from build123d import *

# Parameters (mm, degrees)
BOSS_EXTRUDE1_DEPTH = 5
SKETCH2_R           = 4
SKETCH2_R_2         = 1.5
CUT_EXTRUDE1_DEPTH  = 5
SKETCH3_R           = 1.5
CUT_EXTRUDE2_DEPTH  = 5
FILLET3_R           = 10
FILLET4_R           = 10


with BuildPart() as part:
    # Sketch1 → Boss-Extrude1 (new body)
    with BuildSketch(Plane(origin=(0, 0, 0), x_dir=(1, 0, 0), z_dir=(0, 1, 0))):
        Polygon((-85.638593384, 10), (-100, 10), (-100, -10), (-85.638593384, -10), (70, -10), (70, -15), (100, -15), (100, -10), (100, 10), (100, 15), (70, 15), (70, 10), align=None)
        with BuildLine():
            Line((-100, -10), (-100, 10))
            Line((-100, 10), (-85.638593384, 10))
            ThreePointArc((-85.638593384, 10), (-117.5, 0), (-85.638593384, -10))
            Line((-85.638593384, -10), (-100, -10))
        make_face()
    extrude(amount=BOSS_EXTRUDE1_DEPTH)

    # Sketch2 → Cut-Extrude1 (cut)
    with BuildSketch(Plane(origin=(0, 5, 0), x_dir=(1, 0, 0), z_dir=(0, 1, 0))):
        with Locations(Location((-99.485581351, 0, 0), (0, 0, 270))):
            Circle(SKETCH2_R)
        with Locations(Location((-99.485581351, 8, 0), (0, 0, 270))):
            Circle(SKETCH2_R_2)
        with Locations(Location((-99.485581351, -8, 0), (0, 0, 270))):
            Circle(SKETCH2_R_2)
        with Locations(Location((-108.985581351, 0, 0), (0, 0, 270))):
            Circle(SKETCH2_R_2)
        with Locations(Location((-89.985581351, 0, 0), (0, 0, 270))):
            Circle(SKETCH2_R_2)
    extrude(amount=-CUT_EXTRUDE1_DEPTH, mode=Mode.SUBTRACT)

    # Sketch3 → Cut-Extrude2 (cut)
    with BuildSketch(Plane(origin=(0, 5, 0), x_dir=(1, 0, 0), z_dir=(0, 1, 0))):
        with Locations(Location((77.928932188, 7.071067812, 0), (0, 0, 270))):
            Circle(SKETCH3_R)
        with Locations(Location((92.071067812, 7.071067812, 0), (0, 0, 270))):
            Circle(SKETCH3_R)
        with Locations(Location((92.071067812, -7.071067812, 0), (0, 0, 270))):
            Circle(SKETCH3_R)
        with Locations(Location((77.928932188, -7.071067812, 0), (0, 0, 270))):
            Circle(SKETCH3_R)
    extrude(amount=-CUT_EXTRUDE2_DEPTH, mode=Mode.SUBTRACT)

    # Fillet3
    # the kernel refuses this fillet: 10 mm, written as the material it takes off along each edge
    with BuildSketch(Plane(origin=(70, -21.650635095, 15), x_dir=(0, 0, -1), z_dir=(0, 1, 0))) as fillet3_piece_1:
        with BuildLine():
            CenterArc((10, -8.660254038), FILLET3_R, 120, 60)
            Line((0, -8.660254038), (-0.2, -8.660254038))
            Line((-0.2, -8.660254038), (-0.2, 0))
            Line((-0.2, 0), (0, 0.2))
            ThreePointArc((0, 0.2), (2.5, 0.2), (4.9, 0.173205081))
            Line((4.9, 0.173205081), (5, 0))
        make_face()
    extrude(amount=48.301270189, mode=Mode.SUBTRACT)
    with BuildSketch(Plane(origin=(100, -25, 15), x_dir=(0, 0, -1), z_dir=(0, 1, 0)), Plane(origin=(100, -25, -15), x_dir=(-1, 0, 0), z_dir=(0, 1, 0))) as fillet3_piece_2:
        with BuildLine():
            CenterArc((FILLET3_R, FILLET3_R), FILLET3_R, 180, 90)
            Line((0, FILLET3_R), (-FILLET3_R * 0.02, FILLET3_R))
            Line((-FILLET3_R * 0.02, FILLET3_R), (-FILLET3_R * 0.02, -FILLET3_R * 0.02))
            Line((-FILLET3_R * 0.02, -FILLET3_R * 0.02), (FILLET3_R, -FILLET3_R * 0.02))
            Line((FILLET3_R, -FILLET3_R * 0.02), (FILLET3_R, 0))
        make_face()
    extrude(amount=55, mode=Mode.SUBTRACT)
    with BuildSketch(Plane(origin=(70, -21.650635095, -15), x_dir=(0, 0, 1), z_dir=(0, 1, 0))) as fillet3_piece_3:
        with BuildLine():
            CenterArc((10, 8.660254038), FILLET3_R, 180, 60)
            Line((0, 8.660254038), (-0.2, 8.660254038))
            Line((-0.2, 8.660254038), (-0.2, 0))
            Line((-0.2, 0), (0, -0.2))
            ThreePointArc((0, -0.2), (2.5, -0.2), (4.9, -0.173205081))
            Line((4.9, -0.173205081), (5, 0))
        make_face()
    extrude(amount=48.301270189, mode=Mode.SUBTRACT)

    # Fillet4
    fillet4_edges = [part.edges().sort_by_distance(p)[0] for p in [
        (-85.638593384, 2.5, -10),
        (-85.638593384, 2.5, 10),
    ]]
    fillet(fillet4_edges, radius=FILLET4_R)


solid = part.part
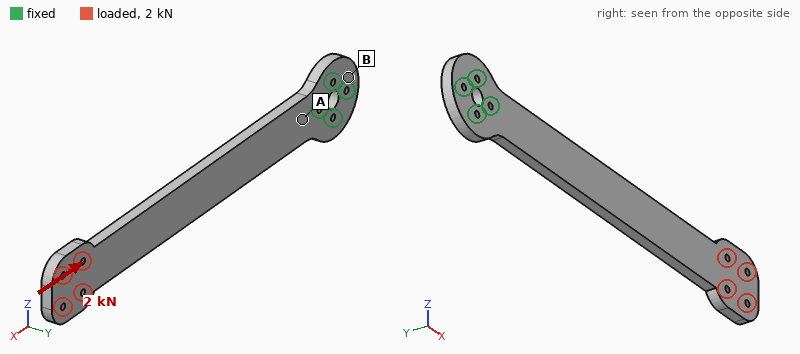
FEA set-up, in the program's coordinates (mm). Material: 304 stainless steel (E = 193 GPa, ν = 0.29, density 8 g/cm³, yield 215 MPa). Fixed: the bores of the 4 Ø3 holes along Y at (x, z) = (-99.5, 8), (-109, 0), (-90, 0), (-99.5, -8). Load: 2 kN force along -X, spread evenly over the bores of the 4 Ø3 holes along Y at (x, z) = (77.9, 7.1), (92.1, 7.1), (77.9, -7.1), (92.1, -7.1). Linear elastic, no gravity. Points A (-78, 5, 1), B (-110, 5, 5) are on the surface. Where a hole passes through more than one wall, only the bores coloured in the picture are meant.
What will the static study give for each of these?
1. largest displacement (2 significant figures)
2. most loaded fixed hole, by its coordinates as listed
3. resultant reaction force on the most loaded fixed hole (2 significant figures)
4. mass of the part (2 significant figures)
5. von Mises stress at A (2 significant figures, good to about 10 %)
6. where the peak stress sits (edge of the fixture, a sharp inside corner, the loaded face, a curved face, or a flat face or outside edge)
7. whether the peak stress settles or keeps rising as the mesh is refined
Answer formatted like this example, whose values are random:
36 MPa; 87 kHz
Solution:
18 µm; (-90, 0); 1.2 kN; 190 g; 21 MPa; edge of the fixture; keeps rising
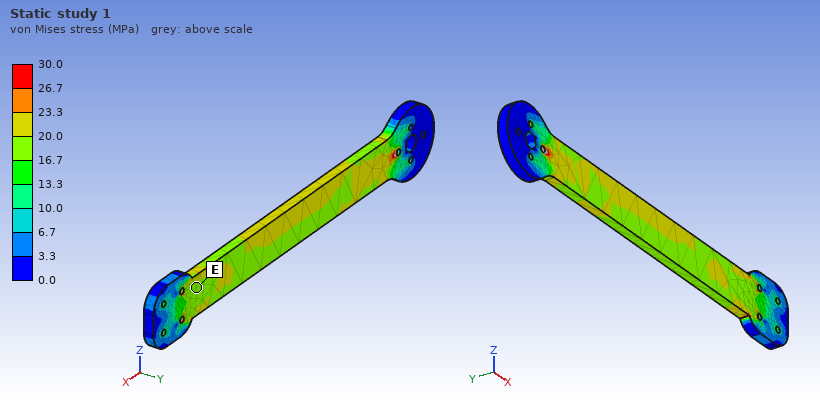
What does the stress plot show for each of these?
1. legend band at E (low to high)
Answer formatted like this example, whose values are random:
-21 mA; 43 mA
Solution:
16.7 to 20.0 MPa
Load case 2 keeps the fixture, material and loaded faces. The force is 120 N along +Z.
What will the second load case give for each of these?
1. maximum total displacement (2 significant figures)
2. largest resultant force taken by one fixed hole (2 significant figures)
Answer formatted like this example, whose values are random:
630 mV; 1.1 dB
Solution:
0.39 mm; 940 N
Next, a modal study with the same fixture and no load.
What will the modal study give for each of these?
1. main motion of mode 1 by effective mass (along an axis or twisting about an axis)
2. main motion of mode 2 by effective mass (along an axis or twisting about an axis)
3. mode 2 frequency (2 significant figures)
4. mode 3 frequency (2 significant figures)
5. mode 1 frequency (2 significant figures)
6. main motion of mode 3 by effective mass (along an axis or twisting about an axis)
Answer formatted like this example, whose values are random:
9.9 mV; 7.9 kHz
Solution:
along Y; along Z; 400 Hz; 670 Hz; 100 Hz; along Y
